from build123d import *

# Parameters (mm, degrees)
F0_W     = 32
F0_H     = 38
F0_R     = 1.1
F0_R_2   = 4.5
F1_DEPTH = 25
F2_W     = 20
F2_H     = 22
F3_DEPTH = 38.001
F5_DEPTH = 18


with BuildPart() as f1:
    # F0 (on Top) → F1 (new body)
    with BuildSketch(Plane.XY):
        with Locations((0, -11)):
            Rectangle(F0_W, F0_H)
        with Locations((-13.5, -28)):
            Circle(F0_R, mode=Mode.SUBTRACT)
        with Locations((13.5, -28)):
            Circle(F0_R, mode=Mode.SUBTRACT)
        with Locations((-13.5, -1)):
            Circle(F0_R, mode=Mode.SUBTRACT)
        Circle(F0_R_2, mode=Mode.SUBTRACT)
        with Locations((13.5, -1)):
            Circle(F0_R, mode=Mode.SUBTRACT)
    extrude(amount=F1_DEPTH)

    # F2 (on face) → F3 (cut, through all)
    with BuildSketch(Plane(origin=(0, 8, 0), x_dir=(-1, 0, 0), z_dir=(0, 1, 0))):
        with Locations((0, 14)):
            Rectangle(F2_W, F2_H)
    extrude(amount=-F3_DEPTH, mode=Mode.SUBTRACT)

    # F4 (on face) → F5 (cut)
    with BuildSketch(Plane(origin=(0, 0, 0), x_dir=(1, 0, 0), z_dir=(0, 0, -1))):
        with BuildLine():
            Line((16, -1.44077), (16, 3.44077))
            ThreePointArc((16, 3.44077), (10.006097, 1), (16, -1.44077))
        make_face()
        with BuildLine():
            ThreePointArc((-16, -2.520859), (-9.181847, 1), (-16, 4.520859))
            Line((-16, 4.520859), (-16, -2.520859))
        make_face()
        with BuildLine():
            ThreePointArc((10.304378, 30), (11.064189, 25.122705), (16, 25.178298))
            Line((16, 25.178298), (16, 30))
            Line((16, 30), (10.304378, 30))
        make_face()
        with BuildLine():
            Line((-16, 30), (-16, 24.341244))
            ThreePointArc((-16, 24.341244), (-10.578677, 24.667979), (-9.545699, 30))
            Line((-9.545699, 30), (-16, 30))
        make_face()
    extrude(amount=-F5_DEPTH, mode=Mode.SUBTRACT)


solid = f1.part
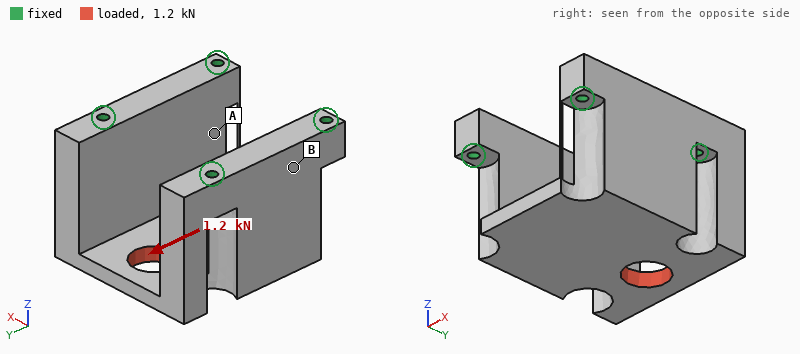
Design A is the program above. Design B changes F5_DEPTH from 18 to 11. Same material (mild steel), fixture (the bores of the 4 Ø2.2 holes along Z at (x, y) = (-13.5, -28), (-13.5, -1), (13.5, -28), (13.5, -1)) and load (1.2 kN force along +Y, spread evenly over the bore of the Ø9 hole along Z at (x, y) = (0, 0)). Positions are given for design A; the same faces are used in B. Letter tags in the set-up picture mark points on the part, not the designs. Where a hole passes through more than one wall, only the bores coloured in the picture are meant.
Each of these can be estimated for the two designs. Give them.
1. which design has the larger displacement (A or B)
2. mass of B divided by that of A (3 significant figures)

A
1.09
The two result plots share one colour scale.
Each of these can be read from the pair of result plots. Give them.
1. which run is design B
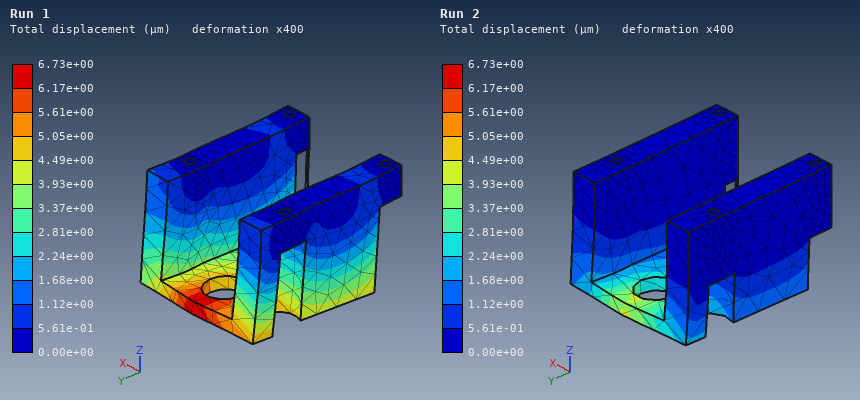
Run 2
